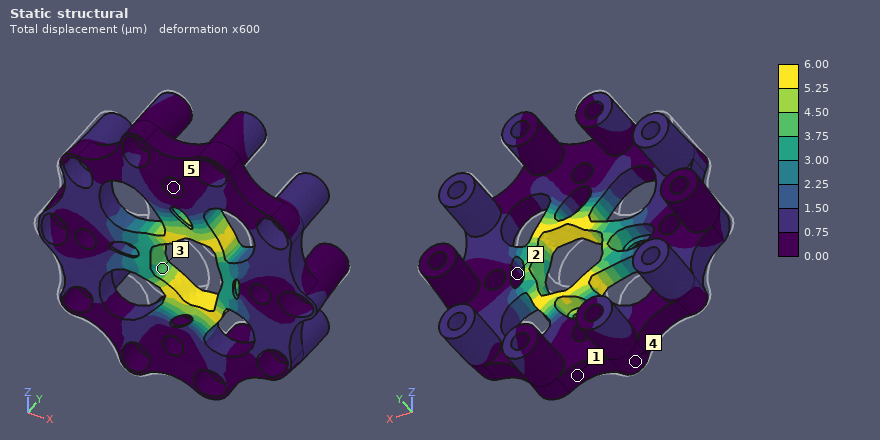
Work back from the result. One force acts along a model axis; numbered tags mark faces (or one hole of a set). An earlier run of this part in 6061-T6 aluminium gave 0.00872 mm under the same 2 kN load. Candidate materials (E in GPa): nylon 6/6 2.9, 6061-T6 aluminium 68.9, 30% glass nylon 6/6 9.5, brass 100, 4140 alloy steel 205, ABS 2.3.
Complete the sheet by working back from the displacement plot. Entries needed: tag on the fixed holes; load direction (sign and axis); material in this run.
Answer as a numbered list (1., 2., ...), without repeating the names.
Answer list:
1. 5
2. +X
3. brass
